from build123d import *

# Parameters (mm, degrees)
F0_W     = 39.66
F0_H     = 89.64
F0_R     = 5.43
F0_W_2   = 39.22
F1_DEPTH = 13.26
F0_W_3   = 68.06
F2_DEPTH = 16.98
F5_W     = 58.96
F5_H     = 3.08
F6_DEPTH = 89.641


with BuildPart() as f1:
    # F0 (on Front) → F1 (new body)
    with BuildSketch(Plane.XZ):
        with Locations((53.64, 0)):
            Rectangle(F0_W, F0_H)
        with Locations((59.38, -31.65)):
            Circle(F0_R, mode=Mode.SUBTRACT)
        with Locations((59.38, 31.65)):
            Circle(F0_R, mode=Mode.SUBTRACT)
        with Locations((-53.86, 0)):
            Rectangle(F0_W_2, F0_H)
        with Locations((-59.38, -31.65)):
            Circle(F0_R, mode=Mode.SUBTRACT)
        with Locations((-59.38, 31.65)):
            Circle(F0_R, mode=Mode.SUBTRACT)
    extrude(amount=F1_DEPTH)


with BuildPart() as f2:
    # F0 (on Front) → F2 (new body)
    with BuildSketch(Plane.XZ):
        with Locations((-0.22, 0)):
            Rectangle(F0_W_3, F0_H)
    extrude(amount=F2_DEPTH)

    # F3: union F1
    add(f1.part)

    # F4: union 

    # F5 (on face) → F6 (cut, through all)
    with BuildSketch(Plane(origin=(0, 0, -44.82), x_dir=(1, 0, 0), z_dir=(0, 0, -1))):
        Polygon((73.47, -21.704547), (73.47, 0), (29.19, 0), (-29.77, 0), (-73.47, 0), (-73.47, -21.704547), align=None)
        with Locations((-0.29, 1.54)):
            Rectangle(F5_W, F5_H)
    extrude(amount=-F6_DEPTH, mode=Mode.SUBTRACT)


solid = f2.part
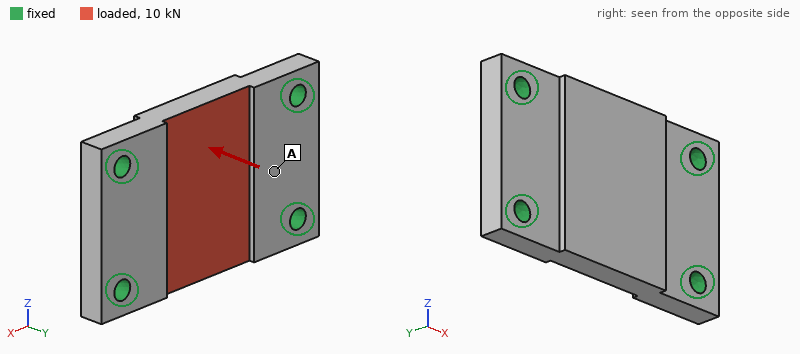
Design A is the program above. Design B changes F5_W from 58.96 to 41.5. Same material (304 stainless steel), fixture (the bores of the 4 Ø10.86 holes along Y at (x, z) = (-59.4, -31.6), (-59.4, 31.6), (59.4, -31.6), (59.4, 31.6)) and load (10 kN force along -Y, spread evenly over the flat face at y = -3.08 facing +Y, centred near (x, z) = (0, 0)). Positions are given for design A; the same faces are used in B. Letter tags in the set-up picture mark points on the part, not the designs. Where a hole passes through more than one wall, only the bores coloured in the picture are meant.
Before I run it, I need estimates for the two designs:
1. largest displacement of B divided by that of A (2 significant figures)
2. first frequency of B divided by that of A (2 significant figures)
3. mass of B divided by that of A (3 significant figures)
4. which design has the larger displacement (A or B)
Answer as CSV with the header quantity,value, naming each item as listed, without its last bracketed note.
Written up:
quantity,value
largest displacement of B divided by that of A,1.1
first frequency of B divided by that of A,0.98
mass of B divided by that of A,1.03
which design has the larger displacement,B
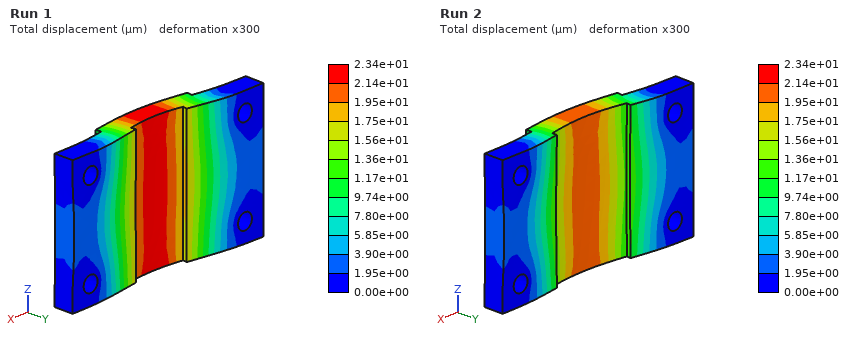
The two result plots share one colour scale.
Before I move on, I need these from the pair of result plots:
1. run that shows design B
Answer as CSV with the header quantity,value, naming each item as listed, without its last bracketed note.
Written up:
quantity,value
run that shows design B,Run 1
